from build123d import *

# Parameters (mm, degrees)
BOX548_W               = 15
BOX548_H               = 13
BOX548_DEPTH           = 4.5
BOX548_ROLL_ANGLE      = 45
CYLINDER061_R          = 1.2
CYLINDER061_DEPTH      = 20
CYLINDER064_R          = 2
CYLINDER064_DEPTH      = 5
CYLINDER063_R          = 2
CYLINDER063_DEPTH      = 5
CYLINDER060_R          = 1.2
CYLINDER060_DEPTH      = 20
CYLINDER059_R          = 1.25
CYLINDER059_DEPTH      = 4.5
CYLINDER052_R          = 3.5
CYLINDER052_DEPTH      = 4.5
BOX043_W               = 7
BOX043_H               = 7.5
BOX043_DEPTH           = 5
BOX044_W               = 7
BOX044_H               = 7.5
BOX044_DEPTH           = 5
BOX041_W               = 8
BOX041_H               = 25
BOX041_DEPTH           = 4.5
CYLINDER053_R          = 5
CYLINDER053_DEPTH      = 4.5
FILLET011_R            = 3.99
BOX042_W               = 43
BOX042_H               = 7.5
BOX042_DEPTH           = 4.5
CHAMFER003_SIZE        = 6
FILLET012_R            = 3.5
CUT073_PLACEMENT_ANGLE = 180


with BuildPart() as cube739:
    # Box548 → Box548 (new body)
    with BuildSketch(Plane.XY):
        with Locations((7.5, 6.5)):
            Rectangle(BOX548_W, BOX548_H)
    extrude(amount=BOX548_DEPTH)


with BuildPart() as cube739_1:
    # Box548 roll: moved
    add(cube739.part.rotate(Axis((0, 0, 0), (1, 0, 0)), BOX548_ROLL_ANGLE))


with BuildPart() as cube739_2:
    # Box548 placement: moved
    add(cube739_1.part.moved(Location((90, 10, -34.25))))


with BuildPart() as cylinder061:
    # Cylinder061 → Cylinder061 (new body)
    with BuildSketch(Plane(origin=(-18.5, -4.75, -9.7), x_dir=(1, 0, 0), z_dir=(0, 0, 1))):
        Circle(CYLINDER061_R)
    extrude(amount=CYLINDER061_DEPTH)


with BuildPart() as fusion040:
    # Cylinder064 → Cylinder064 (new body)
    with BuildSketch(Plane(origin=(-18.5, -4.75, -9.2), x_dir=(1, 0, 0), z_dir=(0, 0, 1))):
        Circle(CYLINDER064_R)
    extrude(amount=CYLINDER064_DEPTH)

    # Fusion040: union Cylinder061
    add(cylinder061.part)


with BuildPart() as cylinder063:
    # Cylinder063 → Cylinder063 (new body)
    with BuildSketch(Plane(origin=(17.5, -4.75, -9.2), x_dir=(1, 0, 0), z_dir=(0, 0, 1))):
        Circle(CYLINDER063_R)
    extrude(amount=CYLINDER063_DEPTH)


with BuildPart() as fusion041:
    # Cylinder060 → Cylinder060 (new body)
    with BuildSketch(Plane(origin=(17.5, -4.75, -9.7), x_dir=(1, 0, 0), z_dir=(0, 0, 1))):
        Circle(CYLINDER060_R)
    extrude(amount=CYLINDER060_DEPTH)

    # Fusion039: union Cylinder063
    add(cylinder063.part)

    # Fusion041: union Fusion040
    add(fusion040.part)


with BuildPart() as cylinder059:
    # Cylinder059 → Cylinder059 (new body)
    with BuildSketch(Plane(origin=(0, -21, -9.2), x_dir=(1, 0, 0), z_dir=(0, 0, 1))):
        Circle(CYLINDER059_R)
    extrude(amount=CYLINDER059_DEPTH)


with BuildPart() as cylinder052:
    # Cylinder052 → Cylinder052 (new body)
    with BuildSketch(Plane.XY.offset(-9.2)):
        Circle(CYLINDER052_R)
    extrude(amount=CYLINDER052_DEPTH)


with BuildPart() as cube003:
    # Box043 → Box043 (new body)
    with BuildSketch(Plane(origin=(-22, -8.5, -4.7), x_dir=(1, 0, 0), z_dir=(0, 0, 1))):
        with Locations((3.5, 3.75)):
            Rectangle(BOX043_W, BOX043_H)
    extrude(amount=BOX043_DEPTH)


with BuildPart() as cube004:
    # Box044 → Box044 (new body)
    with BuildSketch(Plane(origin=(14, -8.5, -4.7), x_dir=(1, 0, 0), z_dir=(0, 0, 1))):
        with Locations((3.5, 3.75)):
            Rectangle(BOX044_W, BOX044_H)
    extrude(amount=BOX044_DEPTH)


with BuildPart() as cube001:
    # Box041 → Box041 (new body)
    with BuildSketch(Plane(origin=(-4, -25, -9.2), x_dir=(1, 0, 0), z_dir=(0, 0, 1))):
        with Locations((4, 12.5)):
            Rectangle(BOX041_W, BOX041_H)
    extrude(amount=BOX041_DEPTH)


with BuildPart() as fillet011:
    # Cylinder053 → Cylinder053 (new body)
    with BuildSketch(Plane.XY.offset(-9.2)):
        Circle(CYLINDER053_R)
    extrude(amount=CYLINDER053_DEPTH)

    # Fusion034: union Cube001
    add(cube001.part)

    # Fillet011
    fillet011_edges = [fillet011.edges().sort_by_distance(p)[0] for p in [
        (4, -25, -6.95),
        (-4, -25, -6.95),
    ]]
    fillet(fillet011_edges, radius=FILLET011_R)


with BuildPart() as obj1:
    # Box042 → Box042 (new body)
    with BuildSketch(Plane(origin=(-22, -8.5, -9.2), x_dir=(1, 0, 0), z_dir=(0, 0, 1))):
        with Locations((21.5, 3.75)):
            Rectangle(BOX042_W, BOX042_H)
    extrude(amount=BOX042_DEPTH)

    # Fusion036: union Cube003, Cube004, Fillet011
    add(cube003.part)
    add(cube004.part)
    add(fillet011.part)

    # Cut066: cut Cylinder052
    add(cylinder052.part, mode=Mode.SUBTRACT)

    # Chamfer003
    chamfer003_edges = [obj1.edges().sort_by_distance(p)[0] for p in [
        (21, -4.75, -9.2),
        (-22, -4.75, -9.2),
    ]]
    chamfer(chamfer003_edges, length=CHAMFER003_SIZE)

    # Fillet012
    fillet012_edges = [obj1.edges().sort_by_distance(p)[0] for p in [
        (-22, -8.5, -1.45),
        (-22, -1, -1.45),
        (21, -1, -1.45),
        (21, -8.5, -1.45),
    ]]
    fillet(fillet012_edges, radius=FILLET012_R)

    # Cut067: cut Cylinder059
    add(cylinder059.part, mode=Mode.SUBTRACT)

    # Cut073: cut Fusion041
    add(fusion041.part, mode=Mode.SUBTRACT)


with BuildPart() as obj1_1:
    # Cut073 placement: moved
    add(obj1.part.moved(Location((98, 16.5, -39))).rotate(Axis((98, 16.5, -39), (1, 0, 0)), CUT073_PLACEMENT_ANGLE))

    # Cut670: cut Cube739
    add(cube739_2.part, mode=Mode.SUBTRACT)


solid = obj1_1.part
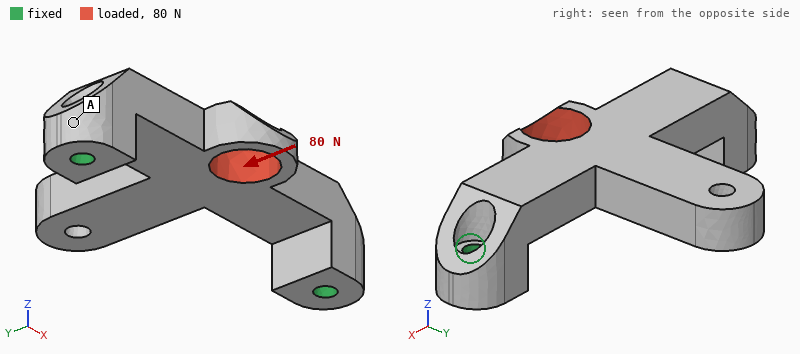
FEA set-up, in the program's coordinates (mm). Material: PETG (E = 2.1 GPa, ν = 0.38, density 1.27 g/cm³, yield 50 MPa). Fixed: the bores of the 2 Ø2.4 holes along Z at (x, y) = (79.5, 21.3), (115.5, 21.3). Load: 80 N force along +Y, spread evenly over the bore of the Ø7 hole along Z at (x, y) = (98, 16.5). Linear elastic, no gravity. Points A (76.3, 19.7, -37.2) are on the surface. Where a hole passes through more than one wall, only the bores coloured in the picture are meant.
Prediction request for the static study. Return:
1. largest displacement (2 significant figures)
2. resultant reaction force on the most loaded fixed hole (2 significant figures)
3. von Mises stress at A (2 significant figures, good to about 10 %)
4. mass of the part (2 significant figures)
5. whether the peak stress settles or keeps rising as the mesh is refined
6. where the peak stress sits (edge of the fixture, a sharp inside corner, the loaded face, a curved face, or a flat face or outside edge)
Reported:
0.15 mm
42 N
2.0 MPa
2.7 g
keeps rising
edge of the fixture
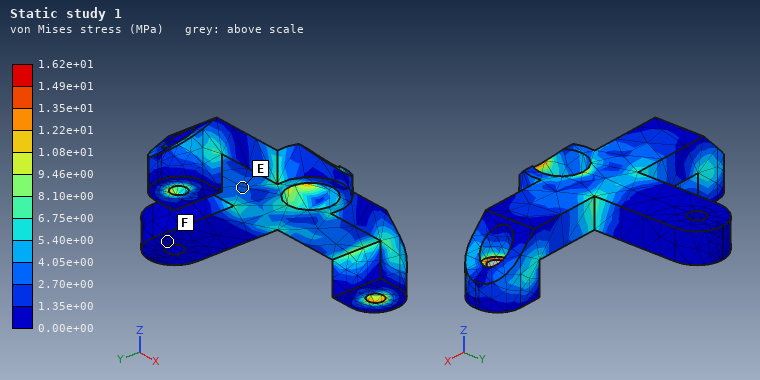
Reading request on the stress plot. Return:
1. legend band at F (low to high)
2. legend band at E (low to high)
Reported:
0.00e+00 to 1.35e+00 MPa
2.70e+00 to 4.05e+00 MPa
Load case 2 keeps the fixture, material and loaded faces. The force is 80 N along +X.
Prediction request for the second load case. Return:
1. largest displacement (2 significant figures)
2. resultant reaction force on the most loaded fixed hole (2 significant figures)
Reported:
0.12 mm
42 N
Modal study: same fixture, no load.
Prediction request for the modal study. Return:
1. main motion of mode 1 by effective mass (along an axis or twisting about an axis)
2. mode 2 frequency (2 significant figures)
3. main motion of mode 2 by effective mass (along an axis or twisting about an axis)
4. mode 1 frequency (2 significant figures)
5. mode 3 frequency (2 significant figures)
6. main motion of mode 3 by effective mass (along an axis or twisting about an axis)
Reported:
along Z
3000 Hz
along Y
1400 Hz
3500 Hz
along X
